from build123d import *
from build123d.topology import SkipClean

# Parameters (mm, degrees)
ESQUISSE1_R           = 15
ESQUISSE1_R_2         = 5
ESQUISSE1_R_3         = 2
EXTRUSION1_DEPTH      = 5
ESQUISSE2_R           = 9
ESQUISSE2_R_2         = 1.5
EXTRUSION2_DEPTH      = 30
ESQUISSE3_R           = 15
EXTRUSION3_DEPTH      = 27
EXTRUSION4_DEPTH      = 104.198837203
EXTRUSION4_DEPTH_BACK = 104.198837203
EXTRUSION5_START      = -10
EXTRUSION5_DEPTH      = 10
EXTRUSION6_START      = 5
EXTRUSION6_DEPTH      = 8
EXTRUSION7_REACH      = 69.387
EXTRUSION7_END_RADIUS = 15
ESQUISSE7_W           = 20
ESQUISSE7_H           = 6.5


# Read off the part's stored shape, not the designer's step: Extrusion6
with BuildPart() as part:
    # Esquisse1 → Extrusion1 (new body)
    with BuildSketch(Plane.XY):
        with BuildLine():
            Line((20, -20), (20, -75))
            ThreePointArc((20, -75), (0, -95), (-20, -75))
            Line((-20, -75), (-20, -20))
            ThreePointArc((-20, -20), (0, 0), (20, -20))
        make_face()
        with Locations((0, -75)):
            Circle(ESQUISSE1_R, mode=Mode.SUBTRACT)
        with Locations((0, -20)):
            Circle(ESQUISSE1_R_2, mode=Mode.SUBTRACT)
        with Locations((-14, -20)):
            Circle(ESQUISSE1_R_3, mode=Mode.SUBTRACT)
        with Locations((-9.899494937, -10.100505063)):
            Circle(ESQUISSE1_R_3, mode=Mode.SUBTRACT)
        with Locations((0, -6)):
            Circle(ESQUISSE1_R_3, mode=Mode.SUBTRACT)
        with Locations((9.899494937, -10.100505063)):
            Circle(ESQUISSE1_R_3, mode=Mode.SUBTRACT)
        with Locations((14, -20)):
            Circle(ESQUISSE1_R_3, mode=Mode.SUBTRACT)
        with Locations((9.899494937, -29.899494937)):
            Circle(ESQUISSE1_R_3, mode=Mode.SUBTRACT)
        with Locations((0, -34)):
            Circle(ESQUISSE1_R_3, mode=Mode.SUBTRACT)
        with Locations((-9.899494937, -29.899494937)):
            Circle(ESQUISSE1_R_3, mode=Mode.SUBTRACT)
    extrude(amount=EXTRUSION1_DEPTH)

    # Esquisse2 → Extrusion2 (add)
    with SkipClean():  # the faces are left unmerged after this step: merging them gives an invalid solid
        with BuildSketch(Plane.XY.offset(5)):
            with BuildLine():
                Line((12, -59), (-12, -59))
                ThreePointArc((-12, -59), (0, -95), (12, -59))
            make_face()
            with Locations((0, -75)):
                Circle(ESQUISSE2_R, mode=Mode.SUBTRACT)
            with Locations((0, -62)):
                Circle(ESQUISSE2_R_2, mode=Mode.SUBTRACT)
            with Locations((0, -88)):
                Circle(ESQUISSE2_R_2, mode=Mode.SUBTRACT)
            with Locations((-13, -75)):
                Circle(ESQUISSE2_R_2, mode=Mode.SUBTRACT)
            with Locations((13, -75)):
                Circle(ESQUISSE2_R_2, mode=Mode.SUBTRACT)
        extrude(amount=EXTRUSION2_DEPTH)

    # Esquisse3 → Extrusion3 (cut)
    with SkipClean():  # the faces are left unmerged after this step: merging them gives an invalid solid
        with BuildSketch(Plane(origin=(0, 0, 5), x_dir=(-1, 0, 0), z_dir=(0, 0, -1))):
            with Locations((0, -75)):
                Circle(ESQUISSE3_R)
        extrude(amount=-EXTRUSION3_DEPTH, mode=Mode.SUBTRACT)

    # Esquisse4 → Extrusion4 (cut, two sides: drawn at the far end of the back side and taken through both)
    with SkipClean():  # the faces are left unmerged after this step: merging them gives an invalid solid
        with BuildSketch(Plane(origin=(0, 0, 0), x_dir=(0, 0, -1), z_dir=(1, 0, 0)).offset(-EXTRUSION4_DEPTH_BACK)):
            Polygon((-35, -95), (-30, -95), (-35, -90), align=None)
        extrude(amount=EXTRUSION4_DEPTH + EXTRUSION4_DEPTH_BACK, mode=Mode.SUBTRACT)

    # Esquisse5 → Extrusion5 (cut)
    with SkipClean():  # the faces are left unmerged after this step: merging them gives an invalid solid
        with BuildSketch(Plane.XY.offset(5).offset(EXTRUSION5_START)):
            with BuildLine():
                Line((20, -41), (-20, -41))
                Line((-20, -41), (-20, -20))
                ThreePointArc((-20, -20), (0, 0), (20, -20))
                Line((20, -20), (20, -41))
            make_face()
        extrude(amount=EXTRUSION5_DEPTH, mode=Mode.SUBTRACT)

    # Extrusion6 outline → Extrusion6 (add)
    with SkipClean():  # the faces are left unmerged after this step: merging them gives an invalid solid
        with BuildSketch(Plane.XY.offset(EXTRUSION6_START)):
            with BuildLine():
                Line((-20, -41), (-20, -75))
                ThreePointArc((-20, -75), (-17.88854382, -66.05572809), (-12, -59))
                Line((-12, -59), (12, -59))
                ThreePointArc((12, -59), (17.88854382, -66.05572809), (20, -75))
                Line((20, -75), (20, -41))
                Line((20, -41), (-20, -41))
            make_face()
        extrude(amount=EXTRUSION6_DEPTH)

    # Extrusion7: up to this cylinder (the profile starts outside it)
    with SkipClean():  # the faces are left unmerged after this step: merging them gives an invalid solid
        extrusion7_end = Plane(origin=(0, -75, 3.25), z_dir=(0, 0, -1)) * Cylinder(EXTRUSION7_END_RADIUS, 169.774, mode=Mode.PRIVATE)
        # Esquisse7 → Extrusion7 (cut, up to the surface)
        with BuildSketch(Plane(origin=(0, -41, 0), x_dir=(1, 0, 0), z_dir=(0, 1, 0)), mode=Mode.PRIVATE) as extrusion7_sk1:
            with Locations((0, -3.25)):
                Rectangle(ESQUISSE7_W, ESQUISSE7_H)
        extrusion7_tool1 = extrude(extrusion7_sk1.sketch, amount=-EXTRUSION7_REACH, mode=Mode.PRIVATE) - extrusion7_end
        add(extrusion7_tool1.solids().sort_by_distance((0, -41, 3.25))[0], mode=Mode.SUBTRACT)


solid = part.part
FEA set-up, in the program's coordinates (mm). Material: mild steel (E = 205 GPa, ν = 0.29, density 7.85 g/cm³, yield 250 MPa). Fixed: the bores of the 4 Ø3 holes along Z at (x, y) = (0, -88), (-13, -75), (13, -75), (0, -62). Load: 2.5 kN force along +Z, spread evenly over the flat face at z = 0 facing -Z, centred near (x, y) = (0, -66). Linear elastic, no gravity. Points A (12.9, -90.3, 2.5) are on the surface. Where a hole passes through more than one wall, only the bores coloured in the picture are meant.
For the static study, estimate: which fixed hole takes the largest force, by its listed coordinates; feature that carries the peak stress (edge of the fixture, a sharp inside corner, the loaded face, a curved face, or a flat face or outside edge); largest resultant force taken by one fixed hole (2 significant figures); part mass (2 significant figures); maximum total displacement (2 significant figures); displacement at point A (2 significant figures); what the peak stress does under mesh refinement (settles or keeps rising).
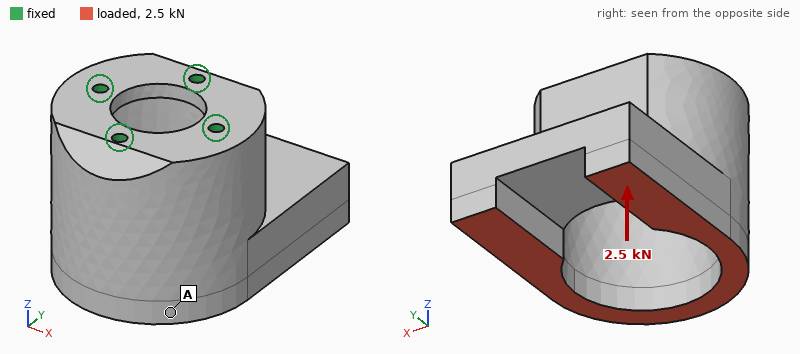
(0, -62)
edge of the fixture
1.2 kN
200 g
20 µm
6.7 µm
keeps rising
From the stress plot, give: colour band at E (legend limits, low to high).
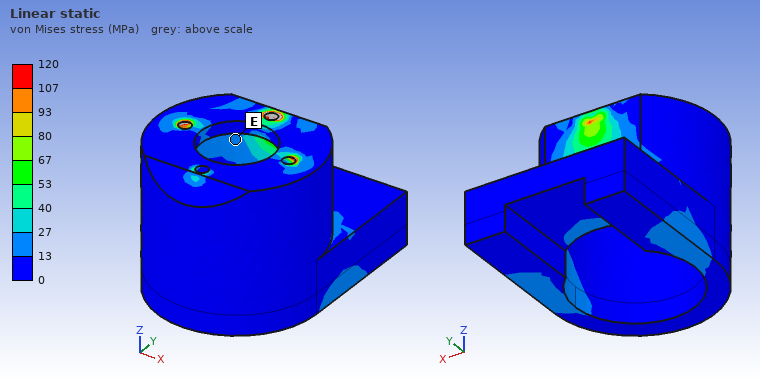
13 to 27 MPa
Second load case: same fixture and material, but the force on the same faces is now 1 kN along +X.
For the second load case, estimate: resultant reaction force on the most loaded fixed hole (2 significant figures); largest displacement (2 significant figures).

1.1 kN
14 µm
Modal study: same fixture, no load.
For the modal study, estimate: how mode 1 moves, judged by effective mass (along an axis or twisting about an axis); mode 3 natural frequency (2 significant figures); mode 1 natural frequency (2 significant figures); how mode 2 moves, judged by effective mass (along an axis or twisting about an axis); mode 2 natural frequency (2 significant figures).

along Y
8800 Hz
4300 Hz
along X
4800 Hz
